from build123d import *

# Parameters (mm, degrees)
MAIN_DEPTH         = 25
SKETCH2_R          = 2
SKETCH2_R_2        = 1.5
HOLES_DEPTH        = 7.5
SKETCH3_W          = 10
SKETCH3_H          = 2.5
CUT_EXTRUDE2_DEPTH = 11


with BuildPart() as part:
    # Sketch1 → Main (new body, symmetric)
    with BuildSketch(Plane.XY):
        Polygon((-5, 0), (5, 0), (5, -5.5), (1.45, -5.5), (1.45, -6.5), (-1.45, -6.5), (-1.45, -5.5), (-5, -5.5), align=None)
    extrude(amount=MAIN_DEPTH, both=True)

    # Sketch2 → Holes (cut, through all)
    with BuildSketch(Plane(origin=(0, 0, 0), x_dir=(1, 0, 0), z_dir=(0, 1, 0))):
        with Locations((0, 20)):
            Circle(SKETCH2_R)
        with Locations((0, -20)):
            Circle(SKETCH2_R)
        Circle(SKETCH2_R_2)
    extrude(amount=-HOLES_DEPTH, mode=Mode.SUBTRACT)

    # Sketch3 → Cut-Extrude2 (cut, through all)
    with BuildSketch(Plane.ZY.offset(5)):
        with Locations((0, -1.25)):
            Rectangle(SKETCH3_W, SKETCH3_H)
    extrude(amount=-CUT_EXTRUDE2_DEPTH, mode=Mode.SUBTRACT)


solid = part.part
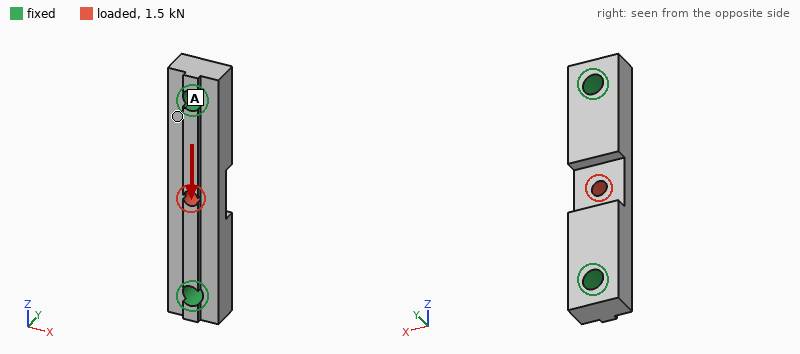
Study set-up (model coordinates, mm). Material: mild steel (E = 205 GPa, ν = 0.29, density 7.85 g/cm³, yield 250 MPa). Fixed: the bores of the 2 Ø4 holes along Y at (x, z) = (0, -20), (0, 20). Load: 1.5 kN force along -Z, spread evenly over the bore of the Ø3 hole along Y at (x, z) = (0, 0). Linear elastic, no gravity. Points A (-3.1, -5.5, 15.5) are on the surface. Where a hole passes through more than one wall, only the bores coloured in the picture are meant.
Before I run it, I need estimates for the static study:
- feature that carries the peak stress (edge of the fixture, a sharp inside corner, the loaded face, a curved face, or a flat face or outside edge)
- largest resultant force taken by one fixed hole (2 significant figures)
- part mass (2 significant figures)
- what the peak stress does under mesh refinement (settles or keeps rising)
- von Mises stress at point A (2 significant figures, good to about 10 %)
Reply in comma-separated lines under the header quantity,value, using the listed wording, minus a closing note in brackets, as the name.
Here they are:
quantity,value
feature that carries the peak stress,a sharp inside corner
largest resultant force taken by one fixed hole,750 N
part mass,19 g
what the peak stress does under mesh refinement,keeps rising
von Mises stress at point A,13 MPa
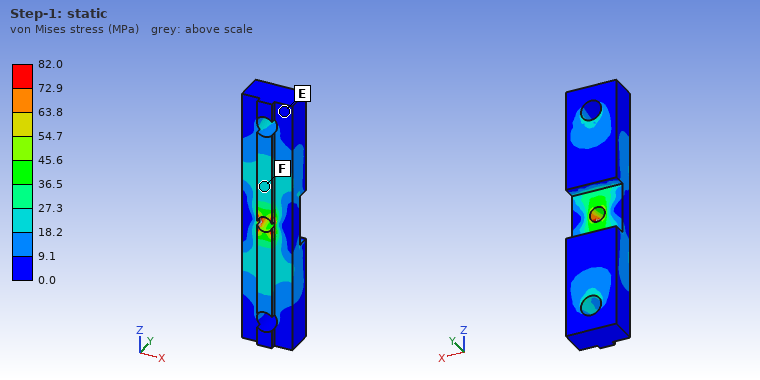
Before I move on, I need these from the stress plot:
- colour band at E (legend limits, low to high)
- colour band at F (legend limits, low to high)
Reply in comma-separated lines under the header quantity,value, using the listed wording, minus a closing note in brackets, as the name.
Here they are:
quantity,value
colour band at E,0.0 to 9.1 MPa
colour band at F,18.2 to 27.3 MPa
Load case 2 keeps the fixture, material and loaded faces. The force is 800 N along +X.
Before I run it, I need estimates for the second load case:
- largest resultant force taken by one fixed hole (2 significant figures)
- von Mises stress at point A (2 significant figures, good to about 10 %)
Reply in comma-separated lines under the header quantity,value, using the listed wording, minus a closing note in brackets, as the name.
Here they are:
quantity,value
largest resultant force taken by one fixed hole,400 N
von Mises stress at point A,25 MPa
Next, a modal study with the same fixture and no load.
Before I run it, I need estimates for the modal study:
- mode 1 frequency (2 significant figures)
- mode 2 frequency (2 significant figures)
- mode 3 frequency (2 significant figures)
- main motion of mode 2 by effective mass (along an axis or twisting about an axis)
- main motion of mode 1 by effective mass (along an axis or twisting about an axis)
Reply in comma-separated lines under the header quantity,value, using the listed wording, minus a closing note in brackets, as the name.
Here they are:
quantity,value
mode 1 frequency,18 kHz
mode 2 frequency,24 kHz
mode 3 frequency,37 kHz
main motion of mode 2 by effective mass,along X
main motion of mode 1 by effective mass,along Y
